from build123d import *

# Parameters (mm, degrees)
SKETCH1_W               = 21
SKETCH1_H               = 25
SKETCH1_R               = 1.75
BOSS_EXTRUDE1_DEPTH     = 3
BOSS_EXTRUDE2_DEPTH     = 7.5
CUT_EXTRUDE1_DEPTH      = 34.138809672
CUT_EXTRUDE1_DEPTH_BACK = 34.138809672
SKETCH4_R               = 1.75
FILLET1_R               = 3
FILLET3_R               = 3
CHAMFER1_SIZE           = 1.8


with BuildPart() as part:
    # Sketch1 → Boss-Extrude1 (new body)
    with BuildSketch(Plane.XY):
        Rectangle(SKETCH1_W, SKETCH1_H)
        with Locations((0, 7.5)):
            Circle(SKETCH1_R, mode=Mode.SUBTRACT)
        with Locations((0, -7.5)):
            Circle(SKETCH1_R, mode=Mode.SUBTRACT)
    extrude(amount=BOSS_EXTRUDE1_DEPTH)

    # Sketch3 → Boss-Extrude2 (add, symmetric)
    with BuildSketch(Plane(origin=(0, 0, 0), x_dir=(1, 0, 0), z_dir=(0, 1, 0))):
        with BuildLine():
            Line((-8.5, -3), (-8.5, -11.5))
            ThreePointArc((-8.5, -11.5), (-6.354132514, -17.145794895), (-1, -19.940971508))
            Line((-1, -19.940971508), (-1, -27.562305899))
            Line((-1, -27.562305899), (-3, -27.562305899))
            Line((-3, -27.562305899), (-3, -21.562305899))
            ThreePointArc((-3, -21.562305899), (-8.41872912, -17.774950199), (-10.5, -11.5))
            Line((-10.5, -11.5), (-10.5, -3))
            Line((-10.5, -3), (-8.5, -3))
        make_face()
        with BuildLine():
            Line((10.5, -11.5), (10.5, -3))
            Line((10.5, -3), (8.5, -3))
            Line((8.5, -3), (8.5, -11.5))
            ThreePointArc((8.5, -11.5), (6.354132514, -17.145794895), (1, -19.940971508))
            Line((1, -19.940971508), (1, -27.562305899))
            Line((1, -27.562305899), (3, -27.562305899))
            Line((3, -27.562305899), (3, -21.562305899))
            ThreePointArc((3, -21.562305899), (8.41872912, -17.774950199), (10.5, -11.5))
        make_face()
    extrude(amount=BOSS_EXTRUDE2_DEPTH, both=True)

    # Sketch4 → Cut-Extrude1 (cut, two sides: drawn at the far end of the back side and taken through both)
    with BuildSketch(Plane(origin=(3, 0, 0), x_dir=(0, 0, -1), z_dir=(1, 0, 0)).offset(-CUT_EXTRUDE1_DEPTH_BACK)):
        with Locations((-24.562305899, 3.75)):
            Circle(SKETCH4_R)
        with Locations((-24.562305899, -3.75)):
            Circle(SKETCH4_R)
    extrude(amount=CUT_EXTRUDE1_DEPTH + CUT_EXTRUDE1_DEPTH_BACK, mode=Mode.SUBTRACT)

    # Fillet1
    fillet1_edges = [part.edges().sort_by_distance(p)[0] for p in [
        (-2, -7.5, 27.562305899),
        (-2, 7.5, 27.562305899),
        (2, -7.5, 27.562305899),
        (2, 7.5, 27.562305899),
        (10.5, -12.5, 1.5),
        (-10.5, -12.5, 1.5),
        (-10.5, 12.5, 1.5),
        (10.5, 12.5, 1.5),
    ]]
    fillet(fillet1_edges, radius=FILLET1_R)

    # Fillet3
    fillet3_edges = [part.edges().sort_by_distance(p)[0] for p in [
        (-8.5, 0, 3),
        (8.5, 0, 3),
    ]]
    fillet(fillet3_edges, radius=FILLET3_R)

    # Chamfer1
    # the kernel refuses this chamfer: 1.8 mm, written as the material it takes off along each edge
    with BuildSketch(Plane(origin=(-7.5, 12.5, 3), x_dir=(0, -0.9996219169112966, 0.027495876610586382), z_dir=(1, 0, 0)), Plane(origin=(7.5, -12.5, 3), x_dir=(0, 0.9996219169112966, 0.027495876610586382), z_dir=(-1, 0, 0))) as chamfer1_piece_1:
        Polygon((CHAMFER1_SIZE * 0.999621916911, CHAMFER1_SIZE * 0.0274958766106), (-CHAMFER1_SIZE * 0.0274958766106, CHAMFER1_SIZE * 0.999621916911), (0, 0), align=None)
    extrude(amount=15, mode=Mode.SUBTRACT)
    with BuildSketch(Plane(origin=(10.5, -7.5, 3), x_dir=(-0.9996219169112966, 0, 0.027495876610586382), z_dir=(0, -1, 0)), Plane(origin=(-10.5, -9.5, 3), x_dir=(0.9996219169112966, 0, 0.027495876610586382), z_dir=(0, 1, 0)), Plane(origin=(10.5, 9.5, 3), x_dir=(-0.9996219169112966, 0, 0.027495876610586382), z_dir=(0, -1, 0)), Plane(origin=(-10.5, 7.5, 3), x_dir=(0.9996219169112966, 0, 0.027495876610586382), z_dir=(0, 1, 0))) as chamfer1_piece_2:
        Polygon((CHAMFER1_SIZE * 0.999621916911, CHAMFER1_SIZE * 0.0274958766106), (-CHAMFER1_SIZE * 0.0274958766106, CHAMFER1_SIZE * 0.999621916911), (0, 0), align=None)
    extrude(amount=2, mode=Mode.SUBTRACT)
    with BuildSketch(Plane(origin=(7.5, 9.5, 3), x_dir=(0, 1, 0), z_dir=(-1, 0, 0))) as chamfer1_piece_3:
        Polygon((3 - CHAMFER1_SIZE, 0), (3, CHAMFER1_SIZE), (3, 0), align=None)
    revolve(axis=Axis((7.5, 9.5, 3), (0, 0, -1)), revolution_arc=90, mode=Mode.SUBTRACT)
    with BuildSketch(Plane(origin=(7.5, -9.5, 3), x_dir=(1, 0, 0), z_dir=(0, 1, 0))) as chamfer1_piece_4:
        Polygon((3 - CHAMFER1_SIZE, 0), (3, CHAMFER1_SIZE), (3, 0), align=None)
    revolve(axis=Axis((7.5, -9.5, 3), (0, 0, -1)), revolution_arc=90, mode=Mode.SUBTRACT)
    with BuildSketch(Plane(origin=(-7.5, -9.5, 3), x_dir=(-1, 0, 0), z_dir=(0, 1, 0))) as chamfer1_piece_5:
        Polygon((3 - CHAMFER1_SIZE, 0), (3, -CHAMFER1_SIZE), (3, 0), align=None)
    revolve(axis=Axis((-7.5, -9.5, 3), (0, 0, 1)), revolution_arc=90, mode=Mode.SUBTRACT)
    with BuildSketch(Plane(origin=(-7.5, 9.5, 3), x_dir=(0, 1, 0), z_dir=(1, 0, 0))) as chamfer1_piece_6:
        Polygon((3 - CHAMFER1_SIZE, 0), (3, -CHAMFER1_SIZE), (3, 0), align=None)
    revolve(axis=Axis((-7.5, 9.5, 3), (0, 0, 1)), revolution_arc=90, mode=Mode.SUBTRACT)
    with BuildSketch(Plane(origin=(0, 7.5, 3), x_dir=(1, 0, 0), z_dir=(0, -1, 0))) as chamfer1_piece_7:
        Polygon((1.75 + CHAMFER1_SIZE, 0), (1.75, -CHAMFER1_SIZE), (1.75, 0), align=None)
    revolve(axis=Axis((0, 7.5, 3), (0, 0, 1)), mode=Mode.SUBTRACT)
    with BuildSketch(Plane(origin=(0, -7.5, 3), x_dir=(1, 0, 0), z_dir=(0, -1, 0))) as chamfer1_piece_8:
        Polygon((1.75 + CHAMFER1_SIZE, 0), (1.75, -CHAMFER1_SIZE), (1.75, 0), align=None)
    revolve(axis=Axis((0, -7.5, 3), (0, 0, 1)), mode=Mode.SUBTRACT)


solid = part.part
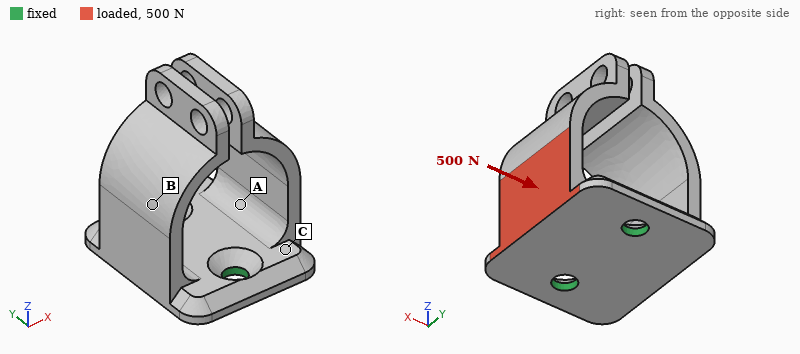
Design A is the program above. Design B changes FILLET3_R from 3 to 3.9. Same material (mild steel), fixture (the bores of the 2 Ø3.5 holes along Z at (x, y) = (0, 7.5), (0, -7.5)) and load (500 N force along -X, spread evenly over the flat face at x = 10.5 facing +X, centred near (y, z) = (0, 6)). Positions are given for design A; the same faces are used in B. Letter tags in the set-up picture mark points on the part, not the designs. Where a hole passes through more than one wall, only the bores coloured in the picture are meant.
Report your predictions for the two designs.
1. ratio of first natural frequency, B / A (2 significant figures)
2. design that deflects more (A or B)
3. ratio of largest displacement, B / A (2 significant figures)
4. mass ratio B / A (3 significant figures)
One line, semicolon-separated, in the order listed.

1.0; A; 0.90; 1.01
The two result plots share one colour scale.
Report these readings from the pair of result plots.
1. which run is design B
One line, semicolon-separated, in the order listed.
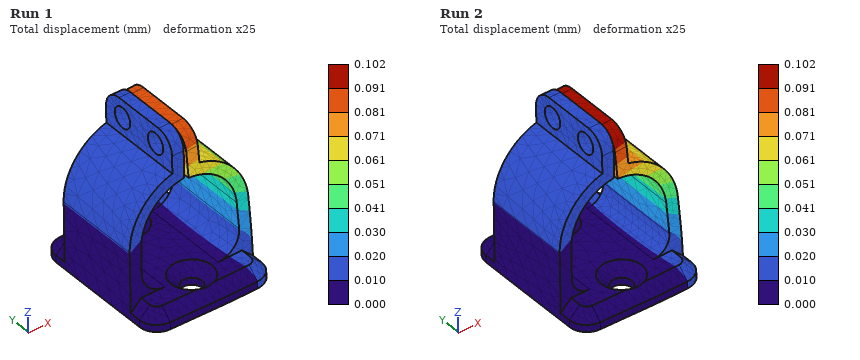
Run 1
